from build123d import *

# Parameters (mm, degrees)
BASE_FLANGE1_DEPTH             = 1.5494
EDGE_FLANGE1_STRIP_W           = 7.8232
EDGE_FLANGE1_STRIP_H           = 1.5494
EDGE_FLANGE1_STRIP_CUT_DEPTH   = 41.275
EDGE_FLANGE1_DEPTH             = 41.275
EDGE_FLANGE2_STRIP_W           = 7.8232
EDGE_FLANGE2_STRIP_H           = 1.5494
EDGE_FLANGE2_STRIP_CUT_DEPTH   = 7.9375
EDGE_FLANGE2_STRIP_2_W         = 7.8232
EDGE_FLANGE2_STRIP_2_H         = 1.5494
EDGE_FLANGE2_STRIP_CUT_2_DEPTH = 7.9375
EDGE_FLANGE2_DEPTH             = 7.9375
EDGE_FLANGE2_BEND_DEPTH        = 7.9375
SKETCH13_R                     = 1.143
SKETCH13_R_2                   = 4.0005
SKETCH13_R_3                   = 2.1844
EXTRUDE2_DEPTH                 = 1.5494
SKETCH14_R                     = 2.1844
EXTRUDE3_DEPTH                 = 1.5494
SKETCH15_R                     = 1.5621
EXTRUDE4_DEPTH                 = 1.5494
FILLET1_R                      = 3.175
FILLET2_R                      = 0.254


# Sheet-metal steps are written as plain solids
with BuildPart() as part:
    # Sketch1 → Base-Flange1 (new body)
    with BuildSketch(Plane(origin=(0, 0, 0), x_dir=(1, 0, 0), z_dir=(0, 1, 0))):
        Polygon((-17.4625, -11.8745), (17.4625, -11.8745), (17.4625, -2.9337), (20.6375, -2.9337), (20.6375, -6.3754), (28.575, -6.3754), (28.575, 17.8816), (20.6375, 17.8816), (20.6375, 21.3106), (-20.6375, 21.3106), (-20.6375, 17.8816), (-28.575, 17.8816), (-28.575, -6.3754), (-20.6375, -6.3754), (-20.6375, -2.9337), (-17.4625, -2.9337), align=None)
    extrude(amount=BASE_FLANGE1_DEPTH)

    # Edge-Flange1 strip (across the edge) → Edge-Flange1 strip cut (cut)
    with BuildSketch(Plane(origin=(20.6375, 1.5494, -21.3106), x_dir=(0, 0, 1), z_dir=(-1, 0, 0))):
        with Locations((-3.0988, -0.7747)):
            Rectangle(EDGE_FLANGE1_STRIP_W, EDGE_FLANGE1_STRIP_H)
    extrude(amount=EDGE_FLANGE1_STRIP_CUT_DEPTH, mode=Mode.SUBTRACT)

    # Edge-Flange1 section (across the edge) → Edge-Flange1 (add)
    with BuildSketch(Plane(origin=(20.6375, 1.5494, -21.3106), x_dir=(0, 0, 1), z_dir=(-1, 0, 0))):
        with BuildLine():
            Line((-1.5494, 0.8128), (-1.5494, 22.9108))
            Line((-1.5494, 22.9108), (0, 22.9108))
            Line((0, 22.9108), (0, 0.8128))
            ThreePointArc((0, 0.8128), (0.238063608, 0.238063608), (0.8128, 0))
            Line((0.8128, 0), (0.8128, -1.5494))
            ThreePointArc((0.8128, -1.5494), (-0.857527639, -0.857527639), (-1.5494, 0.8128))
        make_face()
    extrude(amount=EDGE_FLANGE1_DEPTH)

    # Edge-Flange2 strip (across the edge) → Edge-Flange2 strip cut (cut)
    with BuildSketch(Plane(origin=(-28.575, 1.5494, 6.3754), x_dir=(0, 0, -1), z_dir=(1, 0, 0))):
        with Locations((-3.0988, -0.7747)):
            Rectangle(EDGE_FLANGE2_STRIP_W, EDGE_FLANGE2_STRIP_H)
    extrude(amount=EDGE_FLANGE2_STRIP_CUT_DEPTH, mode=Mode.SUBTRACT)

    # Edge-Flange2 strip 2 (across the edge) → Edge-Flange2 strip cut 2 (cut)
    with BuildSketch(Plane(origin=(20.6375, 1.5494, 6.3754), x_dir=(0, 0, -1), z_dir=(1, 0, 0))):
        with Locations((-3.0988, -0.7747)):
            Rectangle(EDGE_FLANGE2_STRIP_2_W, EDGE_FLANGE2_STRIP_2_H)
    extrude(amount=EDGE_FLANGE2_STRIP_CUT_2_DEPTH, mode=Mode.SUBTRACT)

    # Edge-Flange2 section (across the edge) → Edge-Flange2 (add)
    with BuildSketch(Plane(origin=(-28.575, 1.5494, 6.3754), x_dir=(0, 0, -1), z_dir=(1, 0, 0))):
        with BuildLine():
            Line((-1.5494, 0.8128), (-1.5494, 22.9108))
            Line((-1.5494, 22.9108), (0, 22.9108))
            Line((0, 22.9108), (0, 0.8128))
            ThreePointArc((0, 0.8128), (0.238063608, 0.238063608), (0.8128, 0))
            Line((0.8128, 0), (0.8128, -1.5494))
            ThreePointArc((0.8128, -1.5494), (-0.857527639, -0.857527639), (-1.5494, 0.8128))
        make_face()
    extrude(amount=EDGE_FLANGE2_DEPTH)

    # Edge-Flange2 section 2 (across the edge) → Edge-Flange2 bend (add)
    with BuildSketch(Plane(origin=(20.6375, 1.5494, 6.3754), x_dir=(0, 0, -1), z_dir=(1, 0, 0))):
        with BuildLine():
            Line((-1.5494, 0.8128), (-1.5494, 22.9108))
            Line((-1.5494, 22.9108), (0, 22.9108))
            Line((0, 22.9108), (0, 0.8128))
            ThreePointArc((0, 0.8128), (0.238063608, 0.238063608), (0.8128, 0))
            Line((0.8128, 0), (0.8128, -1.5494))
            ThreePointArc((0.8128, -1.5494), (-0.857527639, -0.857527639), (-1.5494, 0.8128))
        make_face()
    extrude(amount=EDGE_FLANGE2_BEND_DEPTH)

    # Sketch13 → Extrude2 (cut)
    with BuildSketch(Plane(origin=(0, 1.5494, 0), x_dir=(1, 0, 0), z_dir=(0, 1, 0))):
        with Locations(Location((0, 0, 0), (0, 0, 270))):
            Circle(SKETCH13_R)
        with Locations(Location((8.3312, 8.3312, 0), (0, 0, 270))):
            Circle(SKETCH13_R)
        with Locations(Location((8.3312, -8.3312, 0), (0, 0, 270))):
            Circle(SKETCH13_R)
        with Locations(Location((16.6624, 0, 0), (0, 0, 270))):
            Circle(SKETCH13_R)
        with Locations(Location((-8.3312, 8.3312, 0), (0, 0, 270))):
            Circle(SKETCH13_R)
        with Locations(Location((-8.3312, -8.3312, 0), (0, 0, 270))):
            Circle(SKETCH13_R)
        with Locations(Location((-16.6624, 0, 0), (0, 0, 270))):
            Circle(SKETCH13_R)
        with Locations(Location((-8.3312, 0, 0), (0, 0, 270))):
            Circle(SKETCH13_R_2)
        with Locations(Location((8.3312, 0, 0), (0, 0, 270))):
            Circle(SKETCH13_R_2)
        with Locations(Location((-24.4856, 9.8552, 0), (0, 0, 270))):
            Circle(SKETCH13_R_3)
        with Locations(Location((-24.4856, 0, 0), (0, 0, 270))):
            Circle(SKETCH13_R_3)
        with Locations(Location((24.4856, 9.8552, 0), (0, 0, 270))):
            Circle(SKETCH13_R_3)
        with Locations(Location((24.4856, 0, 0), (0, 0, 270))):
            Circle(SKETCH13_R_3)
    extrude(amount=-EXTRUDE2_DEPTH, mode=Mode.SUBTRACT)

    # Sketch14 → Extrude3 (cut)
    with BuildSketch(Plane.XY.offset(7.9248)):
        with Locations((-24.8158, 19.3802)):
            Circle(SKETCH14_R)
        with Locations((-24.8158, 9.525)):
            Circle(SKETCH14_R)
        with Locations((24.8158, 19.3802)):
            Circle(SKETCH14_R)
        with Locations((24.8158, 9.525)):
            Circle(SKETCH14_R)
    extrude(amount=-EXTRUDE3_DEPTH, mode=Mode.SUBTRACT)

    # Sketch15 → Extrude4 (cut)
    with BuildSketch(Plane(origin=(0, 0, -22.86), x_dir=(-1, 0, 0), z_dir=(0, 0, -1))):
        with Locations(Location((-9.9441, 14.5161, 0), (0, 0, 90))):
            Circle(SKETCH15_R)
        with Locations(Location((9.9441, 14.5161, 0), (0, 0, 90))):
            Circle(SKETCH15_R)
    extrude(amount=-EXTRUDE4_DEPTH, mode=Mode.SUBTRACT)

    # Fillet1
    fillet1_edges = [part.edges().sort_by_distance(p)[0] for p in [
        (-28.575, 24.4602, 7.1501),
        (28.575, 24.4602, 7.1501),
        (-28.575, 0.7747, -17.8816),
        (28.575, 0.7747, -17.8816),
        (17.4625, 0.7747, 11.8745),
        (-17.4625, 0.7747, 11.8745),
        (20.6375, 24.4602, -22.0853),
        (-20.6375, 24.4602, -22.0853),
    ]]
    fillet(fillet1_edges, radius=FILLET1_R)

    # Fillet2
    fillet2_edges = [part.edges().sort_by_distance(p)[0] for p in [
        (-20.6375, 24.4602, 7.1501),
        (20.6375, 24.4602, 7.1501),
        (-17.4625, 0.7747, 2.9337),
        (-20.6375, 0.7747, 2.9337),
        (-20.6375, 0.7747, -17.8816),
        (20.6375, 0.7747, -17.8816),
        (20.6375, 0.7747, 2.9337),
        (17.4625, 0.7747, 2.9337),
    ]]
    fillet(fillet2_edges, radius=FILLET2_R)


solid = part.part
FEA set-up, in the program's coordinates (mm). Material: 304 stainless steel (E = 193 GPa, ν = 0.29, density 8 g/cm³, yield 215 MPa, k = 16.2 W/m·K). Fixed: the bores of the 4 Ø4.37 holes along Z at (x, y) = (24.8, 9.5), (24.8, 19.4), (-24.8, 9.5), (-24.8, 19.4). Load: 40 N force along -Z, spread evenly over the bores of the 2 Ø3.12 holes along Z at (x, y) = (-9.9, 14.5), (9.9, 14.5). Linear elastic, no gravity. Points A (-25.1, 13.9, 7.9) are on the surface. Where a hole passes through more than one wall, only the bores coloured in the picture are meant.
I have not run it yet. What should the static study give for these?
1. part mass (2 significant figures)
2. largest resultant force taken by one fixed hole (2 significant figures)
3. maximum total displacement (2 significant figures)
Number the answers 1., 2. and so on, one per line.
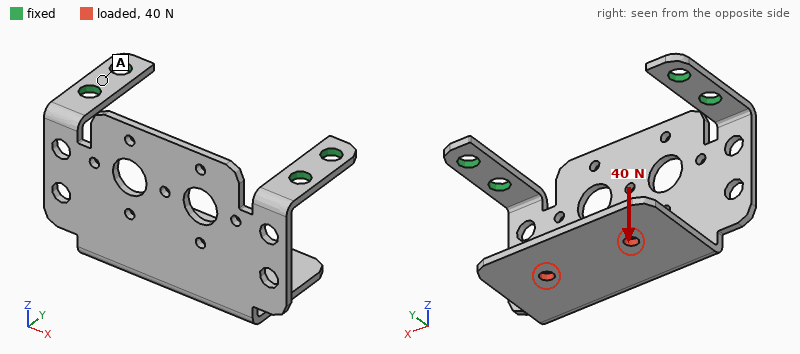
1. 34 g
2. 21 N
3. 0.43 mm
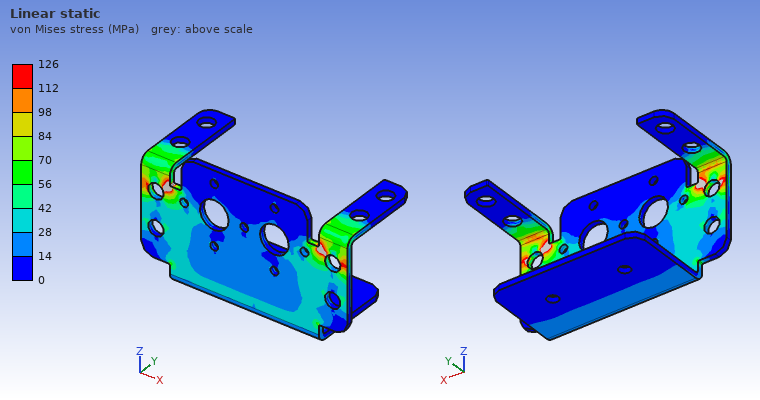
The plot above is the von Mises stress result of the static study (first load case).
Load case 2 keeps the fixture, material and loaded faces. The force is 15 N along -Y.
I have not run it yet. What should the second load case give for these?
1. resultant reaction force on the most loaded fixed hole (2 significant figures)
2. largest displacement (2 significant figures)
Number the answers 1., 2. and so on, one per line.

1. 7.4 N
2. 0.28 mm
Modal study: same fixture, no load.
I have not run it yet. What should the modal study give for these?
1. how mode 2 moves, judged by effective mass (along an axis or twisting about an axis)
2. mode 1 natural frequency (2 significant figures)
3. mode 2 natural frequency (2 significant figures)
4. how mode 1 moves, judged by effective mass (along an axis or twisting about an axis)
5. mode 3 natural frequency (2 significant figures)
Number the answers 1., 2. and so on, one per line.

1. along X
2. 300 Hz
3. 980 Hz
4. along Y
5. 1300 Hz
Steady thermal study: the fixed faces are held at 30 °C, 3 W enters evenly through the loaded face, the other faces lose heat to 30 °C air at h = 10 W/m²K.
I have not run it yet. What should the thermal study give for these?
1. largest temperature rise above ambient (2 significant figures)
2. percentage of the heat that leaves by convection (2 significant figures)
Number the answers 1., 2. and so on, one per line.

1. 86 K
2. 82 %
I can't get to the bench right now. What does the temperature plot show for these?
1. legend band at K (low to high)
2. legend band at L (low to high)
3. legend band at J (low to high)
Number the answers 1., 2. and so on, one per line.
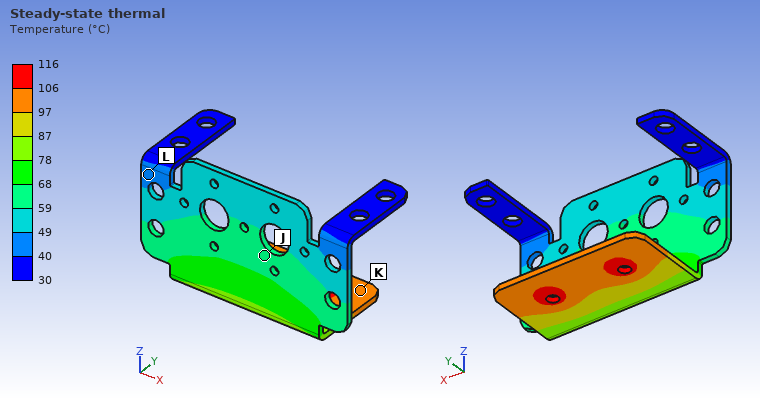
1. 97 to 106 °C
2. 40 to 49 °C
3. 59 to 68 °C
